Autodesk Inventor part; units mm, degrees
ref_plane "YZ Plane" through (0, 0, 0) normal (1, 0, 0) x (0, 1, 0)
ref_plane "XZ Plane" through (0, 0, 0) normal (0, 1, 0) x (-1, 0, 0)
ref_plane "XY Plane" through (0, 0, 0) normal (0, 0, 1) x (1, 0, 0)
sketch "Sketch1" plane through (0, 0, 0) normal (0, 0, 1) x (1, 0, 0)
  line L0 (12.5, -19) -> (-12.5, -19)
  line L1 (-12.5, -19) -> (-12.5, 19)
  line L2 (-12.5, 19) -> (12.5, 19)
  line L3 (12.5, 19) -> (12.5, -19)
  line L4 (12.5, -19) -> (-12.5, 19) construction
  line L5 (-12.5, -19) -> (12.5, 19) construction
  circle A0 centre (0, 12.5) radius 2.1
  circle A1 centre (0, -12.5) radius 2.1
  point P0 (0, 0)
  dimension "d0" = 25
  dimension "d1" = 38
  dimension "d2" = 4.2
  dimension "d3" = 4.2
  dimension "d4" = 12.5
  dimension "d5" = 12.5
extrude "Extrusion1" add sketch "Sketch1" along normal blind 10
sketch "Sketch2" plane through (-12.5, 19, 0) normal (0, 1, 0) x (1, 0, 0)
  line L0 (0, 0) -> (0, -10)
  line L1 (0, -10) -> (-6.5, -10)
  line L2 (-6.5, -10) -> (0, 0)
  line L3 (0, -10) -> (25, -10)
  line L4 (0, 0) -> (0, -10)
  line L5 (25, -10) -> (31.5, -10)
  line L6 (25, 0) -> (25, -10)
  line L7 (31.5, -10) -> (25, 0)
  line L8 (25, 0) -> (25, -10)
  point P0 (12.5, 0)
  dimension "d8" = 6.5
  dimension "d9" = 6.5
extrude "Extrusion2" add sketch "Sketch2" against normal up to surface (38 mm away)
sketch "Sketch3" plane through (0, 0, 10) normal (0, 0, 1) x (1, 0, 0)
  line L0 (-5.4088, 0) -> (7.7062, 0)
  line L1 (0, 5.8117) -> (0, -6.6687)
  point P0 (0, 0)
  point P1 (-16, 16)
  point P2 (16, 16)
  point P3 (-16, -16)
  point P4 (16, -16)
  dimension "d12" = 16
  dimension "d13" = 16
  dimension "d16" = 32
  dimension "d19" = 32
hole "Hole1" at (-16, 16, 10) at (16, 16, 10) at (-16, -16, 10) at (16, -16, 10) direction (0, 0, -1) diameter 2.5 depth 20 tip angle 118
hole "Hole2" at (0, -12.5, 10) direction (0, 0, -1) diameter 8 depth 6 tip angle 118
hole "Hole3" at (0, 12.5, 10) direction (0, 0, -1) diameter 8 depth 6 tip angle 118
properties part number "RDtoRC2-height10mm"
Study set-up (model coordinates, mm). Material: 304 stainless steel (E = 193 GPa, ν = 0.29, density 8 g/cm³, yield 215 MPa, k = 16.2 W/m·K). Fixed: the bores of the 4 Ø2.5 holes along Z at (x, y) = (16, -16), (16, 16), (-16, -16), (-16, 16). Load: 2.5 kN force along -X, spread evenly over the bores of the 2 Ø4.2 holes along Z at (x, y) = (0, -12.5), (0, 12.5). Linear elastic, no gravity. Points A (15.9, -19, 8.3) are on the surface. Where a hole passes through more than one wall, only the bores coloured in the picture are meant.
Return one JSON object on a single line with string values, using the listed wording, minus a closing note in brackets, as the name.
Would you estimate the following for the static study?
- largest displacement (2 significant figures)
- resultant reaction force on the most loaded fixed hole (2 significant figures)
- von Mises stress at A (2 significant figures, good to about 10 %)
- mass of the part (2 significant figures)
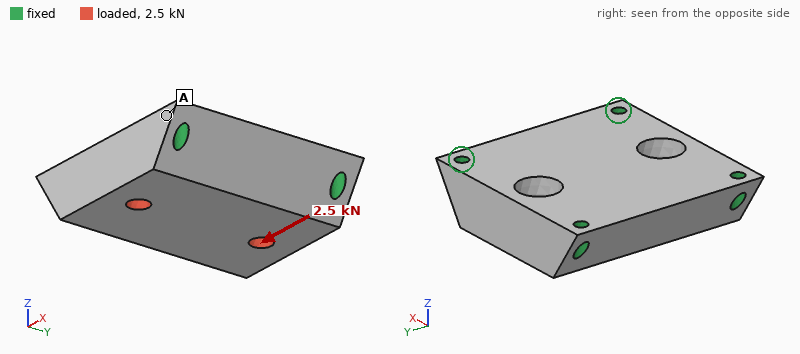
{"largest displacement": "1.5 µm", "resultant reaction force on the most loaded fixed hole": "680 N", "von Mises stress at A": "5.1 MPa", "mass of the part": "89 g"}
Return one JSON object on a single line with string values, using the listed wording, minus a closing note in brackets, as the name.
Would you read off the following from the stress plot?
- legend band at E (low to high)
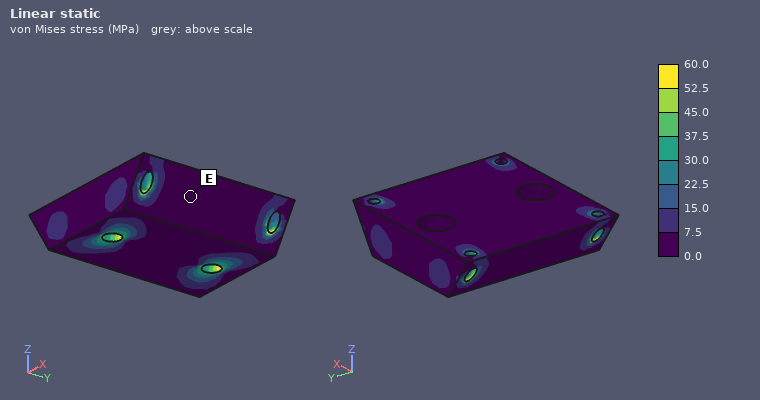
{"legend band at E": "0.0 to 7.5 MPa"}
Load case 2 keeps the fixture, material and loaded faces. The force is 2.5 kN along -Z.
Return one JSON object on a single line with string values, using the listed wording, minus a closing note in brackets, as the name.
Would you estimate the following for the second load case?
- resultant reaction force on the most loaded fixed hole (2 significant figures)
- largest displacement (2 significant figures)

{"resultant reaction force on the most loaded fixed hole": "780 N", "largest displacement": "5.0 µm"}
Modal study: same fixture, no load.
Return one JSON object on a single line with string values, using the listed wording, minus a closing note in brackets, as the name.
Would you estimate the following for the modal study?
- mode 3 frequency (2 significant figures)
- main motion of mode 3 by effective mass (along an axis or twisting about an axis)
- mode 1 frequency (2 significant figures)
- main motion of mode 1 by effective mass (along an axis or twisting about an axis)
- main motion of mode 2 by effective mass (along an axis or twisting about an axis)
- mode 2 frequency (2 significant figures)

{"mode 3 frequency": "30 kHz", "main motion of mode 3 by effective mass": "along Y", "mode 1 frequency": "18 kHz", "main motion of mode 1 by effective mass": "along Z", "main motion of mode 2 by effective mass": "along X", "mode 2 frequency": "27 kHz"}
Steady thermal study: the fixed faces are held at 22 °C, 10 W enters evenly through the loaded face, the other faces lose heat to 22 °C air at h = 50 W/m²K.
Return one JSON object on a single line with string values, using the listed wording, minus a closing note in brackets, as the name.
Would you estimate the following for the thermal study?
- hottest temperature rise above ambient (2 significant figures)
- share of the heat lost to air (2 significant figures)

{"hottest temperature rise above ambient": "34 K", "share of the heat lost to air": "25 %"}
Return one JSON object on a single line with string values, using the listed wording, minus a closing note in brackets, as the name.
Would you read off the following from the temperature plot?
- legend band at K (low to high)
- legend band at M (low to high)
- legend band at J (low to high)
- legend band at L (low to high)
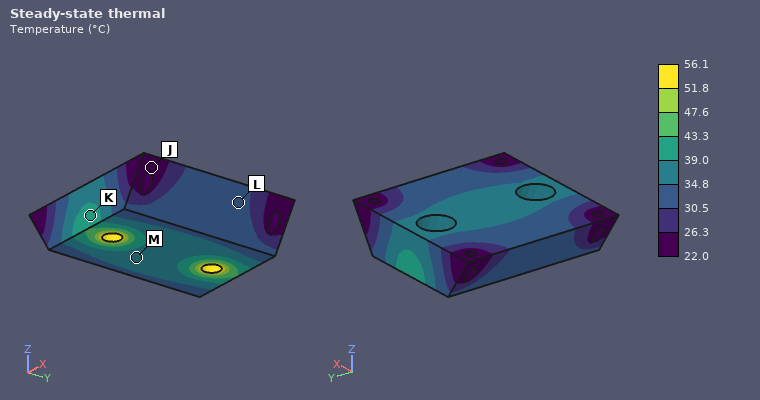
{"legend band at K": "39.0 to 43.3 °C", "legend band at M": "34.8 to 39.0 °C", "legend band at J": "22.0 to 26.3 °C", "legend band at L": "30.5 to 34.8 °C"}
